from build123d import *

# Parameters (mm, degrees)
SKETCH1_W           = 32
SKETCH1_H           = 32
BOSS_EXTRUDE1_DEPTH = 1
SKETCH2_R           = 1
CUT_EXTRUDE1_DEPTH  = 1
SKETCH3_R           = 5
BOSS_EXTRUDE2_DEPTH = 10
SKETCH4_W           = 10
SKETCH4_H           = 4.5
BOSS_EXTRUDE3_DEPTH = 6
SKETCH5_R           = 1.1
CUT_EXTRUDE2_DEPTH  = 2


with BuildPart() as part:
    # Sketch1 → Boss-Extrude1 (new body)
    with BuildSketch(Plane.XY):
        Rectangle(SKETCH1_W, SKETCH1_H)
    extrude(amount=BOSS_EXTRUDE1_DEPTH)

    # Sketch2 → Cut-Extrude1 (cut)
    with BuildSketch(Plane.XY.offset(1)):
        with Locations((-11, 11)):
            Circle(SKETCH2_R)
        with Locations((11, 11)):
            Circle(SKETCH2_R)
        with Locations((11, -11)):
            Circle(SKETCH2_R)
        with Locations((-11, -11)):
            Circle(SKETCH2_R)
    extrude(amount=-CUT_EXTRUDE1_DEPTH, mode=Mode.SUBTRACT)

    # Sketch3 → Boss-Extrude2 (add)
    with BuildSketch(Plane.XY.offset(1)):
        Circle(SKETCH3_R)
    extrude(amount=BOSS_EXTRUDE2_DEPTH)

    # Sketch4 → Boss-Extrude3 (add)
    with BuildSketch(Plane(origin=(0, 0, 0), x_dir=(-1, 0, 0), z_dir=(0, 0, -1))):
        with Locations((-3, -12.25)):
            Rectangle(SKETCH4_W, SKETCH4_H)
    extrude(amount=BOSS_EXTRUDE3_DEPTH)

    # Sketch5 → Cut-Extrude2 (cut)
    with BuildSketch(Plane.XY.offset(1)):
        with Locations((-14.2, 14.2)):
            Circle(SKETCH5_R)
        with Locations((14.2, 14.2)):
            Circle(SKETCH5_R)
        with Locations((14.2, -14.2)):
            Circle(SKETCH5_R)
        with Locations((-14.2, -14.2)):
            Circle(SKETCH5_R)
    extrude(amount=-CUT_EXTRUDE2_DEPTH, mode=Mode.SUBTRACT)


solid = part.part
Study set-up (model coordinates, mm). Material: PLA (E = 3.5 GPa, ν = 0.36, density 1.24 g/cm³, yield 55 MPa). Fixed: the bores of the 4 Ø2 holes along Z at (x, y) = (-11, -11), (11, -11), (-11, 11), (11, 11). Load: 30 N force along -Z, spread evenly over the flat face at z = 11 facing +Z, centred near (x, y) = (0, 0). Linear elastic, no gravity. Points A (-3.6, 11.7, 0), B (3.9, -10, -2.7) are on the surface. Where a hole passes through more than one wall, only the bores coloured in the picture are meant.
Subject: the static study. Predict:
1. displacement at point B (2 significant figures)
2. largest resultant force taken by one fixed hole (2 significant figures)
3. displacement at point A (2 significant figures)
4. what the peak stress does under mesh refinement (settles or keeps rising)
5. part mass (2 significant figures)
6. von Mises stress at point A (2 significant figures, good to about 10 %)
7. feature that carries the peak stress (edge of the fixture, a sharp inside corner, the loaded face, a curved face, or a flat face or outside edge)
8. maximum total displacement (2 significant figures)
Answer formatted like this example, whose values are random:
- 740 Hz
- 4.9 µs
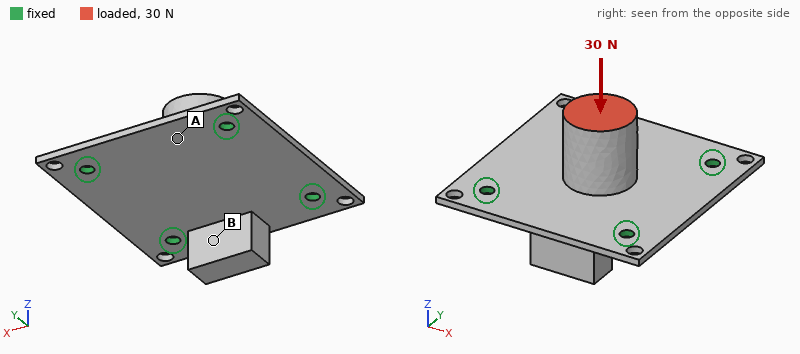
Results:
- 0.085 mm
- 7.9 N
- 0.077 mm
- keeps rising
- 2.5 g
- 5.3 MPa
- edge of the fixture
- 0.21 mm
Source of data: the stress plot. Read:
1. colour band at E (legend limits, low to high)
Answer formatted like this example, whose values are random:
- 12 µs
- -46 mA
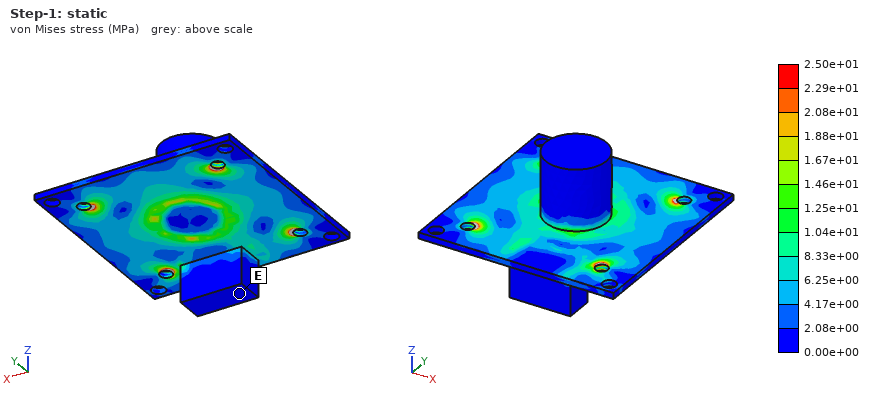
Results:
- 0.00e+00 to 2.08e+00 MPa
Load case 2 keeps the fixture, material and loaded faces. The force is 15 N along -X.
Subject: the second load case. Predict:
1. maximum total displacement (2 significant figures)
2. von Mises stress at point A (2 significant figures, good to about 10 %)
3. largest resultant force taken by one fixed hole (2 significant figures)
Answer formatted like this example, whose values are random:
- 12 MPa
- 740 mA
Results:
- 0.21 mm
- 2.5 MPa
- 6.3 N
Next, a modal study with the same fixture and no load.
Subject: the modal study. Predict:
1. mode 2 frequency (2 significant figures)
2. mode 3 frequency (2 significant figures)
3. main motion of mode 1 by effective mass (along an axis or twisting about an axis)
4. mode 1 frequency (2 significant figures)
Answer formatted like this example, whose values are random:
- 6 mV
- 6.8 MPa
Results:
- 2100 Hz
- 2100 Hz
- along Z
- 1700 Hz
